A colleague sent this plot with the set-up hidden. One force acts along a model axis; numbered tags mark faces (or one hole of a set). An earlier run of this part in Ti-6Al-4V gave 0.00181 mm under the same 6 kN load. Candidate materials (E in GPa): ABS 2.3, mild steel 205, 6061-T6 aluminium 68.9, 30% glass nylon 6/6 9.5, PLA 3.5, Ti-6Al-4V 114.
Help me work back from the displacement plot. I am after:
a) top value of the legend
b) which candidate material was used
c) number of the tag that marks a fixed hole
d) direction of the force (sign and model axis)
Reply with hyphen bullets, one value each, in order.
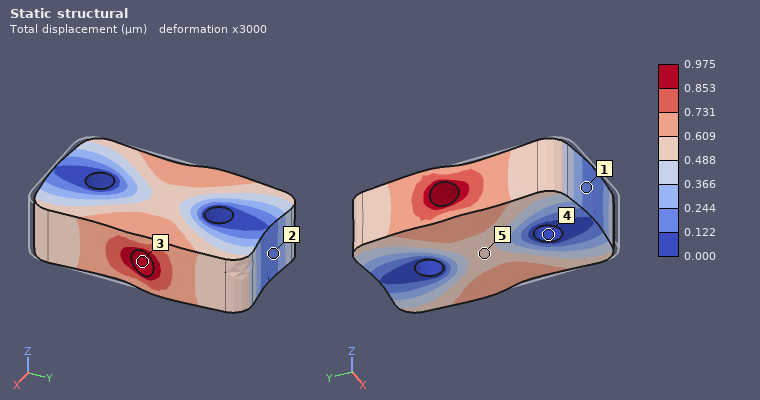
- 0.975 µm
- mild steel
- 4
- +Y
